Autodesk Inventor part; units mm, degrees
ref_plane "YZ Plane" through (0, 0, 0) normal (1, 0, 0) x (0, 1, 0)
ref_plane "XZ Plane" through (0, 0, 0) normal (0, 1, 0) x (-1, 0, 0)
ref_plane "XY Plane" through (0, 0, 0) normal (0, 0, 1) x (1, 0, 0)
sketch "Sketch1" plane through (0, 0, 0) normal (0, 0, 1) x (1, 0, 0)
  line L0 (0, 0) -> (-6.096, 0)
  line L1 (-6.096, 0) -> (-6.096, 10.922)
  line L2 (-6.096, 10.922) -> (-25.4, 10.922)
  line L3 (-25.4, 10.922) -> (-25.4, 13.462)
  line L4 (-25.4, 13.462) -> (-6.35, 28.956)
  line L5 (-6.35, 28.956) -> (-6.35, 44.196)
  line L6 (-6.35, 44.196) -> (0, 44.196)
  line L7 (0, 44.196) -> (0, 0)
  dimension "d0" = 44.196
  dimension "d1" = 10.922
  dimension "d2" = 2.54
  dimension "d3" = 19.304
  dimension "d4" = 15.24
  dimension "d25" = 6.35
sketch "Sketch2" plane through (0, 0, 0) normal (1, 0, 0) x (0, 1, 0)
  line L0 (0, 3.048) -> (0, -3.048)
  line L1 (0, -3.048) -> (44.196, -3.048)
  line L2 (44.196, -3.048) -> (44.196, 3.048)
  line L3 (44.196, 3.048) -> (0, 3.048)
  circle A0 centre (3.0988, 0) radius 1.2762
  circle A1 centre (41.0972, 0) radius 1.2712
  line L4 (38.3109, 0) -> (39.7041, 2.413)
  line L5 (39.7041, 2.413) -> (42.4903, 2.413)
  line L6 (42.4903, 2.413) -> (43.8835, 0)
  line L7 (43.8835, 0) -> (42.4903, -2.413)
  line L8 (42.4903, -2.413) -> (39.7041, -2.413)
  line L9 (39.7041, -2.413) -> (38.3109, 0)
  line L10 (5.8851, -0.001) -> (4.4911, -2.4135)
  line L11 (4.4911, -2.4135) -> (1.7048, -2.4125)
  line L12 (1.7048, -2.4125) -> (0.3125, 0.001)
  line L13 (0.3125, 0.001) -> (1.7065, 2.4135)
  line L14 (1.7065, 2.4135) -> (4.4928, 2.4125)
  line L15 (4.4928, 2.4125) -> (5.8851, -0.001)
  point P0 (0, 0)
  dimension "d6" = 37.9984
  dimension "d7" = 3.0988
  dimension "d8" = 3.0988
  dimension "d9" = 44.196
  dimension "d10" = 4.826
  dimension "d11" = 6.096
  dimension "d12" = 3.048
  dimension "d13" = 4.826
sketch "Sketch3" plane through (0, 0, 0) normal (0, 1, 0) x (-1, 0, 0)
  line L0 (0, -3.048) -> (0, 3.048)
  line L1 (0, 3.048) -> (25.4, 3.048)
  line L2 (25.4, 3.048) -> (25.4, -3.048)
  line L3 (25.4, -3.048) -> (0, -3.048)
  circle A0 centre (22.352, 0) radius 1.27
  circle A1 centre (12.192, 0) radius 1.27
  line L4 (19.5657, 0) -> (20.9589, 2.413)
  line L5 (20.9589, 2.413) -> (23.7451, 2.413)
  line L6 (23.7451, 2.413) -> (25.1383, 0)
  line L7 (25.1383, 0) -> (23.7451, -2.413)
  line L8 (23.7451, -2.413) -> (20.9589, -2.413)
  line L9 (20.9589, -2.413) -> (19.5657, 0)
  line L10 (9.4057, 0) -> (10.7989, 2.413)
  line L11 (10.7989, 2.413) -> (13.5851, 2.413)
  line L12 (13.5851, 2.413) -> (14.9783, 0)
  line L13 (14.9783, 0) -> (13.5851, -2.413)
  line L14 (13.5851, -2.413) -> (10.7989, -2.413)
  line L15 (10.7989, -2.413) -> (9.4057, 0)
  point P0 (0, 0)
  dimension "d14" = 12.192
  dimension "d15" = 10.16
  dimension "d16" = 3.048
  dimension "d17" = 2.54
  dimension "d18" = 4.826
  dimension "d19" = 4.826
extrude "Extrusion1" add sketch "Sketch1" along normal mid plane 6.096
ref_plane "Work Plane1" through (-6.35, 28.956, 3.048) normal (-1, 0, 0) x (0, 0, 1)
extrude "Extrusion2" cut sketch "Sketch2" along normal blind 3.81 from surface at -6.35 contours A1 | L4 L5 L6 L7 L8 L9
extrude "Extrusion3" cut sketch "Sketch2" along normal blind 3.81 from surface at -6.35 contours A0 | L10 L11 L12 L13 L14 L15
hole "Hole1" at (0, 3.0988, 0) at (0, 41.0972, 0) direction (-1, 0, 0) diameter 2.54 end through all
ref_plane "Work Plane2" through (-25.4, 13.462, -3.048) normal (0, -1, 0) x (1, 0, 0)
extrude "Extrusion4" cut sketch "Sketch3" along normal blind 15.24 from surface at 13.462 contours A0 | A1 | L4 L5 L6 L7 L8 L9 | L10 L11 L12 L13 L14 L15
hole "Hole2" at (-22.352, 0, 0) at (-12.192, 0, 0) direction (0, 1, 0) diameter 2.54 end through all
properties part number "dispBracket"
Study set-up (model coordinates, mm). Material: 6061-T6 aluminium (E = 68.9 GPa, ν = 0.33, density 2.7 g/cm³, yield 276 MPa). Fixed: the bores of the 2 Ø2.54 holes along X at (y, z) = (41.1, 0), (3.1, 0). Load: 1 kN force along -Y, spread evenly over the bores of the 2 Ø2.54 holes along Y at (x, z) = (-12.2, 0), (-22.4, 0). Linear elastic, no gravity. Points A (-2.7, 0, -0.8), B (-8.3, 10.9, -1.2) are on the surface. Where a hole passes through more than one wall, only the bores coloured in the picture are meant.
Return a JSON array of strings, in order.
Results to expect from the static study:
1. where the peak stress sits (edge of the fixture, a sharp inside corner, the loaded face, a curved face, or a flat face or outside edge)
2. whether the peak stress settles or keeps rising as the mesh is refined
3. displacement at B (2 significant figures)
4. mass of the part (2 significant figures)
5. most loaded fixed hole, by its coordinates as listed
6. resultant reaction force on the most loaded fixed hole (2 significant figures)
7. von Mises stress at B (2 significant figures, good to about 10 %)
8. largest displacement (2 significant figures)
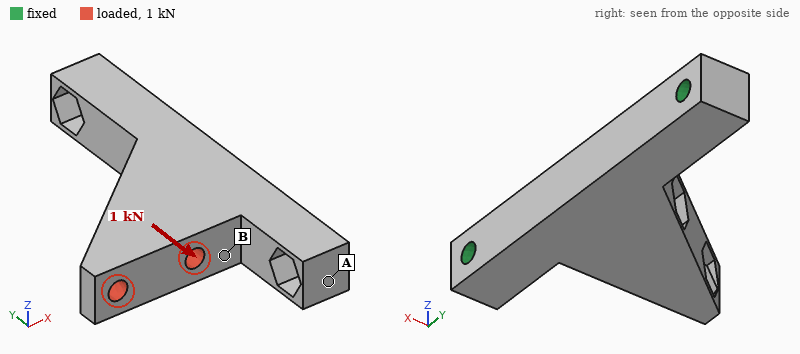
["edge of the fixture", "keeps rising", "14 µm", "6.5 g", "(41.1, 0)", "810 N", "80 MPa", "90 µm"]
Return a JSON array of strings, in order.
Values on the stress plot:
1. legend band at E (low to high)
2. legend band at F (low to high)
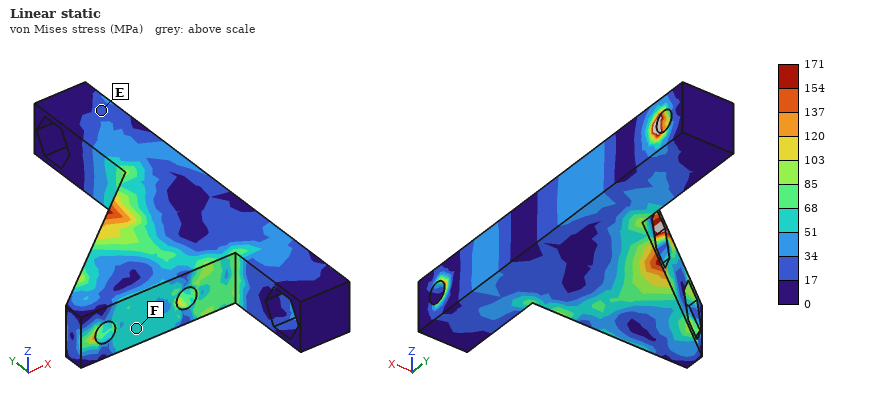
["17 to 34 MPa", "51 to 68 MPa"]
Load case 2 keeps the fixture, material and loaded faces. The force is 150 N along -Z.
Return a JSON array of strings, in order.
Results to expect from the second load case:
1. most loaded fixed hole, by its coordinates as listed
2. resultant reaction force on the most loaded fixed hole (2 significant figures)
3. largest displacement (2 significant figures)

["(3.1, 0)", "120 N", "0.13 mm"]
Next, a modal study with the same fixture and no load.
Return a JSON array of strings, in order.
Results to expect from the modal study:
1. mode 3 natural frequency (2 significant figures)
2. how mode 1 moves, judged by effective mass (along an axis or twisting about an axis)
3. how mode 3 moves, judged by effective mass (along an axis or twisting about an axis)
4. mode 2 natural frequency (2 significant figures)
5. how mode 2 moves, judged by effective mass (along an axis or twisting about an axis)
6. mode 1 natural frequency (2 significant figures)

["15 kHz", "along Z", "along Z", "14 kHz", "along X", "5300 Hz"]
